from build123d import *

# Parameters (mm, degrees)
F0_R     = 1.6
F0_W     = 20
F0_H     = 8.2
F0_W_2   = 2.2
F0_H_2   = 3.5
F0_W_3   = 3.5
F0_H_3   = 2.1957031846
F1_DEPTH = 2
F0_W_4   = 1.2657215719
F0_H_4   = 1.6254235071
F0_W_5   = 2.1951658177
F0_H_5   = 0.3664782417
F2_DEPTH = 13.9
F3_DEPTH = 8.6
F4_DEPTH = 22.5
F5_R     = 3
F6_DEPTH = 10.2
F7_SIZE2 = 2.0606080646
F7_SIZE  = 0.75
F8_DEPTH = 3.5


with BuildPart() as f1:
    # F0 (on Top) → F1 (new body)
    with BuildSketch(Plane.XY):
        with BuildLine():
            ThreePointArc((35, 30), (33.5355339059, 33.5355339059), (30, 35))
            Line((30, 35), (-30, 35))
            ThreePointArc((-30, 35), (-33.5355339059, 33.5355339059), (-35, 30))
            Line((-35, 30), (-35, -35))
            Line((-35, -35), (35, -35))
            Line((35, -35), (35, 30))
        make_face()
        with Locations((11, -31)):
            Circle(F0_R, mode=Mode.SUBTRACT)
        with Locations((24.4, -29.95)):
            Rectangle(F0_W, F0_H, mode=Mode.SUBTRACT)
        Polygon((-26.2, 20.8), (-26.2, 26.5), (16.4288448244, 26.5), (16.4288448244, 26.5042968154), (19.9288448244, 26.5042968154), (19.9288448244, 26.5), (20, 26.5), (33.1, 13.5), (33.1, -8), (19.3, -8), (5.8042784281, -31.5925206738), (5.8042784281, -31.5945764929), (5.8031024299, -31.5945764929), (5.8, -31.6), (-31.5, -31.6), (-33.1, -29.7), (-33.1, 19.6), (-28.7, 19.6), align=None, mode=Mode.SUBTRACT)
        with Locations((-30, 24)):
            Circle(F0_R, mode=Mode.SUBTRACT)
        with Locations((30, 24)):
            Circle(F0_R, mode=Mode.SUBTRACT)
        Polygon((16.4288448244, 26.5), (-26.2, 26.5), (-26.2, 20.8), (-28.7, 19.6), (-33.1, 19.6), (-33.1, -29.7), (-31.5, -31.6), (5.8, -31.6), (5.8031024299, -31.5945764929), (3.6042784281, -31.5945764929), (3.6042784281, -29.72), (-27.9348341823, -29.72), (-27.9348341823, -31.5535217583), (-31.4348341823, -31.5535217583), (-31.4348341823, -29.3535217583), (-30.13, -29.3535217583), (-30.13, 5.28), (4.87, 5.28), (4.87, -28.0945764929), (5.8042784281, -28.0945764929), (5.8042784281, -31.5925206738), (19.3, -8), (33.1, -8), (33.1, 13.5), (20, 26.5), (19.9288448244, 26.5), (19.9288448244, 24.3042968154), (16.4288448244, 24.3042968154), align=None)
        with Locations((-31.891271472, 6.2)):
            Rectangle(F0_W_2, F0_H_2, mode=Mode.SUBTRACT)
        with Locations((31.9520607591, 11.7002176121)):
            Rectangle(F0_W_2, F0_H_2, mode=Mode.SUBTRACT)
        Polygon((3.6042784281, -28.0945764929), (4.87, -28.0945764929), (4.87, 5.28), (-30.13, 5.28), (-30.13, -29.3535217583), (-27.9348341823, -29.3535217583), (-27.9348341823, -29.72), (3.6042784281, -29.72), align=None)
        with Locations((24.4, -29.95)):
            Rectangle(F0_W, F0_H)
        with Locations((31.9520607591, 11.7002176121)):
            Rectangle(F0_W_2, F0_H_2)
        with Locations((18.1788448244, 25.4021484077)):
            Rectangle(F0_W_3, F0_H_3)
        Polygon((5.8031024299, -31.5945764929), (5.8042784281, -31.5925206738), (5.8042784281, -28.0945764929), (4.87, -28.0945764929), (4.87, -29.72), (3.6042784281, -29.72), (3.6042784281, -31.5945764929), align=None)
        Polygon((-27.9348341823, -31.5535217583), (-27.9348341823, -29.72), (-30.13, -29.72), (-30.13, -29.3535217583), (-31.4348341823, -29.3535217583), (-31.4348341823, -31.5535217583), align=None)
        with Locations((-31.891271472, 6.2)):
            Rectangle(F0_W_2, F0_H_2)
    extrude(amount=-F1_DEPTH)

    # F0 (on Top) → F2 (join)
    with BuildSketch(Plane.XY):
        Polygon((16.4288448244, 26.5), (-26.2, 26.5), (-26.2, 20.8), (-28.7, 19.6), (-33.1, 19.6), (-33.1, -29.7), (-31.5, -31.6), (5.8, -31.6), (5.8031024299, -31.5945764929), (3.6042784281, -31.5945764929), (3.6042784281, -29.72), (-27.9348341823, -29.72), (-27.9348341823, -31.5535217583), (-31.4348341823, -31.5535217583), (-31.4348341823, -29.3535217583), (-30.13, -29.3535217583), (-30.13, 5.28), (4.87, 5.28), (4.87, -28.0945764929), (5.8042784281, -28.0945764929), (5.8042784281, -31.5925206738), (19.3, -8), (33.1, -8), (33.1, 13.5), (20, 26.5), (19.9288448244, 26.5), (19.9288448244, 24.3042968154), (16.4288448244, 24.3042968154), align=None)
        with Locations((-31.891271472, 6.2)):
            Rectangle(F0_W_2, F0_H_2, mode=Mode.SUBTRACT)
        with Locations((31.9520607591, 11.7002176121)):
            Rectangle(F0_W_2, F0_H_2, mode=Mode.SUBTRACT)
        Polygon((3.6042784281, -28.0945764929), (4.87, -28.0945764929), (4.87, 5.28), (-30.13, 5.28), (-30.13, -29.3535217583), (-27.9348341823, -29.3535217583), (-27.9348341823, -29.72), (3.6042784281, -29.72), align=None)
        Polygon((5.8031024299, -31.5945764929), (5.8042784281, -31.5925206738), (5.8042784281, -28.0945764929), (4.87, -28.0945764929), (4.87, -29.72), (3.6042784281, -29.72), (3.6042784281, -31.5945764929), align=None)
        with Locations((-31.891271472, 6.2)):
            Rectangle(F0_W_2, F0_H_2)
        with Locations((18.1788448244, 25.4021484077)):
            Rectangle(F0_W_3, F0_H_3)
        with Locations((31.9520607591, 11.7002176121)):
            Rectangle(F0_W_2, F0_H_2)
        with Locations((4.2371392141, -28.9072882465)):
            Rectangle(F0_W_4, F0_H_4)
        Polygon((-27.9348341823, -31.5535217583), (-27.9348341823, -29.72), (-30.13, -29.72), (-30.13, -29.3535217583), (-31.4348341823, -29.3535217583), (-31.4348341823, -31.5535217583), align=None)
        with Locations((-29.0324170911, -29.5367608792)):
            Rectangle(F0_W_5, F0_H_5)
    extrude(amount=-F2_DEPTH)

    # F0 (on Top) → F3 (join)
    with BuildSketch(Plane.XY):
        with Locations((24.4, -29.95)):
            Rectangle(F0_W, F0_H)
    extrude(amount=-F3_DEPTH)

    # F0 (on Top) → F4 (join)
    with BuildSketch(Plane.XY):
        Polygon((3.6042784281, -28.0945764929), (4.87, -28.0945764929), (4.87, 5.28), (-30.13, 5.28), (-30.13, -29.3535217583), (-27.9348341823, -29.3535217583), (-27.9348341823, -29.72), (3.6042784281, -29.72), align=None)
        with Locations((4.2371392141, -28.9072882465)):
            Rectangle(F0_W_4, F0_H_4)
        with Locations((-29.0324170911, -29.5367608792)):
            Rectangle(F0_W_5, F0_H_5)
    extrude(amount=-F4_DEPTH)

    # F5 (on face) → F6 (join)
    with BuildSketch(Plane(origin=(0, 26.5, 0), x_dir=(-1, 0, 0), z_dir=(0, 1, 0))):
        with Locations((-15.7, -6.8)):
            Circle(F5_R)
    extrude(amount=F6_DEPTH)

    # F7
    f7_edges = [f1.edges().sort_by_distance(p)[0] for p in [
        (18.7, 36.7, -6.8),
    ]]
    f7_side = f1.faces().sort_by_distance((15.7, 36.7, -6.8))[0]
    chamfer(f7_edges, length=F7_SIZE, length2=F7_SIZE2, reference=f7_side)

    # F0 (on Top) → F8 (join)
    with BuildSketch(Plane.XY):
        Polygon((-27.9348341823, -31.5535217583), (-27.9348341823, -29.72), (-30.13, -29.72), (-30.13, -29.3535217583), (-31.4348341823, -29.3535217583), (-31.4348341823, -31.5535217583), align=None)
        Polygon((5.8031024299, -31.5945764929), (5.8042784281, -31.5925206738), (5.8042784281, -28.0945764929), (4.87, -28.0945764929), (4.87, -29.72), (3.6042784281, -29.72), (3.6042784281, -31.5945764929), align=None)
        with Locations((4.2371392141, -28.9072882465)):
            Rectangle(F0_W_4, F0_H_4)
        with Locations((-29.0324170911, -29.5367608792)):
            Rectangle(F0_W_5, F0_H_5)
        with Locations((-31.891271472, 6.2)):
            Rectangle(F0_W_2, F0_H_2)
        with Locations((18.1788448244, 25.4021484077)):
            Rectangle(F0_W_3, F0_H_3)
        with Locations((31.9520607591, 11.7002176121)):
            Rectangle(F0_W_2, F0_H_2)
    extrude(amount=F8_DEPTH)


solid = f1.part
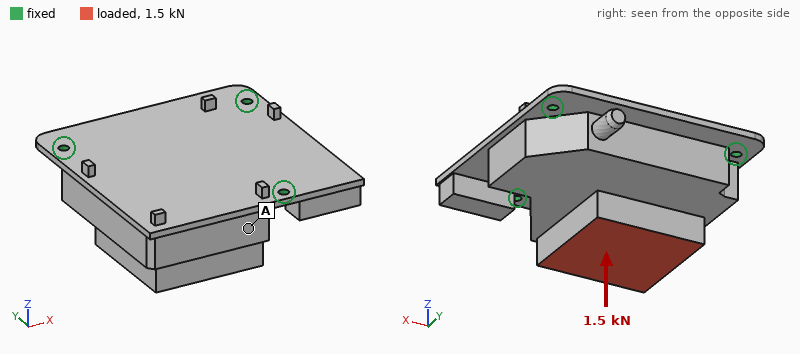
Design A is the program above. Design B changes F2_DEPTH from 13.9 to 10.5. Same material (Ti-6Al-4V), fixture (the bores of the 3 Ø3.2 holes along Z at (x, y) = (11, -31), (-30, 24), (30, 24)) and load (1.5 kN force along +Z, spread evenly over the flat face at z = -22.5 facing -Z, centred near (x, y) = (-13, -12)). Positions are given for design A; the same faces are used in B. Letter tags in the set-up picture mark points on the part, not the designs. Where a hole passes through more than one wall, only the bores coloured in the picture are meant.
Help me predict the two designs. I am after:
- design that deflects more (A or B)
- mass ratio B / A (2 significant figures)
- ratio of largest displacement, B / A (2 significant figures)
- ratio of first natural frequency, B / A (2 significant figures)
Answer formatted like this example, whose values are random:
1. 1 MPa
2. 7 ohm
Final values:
1. B
2. 0.89
3. 1.2
4. 0.95
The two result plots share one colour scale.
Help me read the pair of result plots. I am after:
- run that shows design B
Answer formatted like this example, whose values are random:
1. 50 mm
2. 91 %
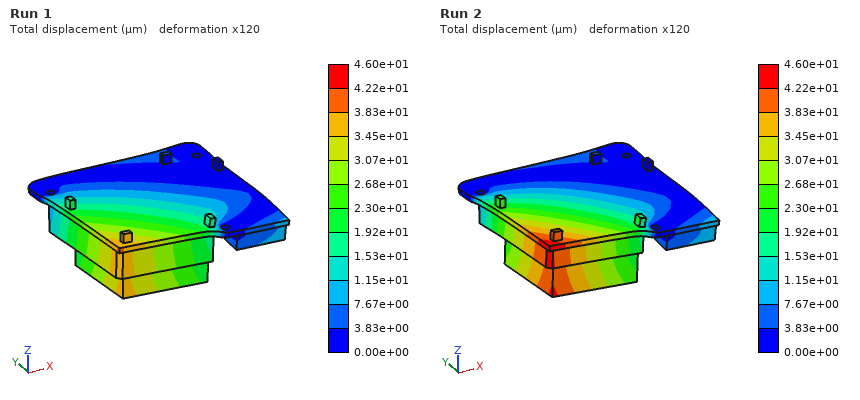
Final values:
1. Run 2
